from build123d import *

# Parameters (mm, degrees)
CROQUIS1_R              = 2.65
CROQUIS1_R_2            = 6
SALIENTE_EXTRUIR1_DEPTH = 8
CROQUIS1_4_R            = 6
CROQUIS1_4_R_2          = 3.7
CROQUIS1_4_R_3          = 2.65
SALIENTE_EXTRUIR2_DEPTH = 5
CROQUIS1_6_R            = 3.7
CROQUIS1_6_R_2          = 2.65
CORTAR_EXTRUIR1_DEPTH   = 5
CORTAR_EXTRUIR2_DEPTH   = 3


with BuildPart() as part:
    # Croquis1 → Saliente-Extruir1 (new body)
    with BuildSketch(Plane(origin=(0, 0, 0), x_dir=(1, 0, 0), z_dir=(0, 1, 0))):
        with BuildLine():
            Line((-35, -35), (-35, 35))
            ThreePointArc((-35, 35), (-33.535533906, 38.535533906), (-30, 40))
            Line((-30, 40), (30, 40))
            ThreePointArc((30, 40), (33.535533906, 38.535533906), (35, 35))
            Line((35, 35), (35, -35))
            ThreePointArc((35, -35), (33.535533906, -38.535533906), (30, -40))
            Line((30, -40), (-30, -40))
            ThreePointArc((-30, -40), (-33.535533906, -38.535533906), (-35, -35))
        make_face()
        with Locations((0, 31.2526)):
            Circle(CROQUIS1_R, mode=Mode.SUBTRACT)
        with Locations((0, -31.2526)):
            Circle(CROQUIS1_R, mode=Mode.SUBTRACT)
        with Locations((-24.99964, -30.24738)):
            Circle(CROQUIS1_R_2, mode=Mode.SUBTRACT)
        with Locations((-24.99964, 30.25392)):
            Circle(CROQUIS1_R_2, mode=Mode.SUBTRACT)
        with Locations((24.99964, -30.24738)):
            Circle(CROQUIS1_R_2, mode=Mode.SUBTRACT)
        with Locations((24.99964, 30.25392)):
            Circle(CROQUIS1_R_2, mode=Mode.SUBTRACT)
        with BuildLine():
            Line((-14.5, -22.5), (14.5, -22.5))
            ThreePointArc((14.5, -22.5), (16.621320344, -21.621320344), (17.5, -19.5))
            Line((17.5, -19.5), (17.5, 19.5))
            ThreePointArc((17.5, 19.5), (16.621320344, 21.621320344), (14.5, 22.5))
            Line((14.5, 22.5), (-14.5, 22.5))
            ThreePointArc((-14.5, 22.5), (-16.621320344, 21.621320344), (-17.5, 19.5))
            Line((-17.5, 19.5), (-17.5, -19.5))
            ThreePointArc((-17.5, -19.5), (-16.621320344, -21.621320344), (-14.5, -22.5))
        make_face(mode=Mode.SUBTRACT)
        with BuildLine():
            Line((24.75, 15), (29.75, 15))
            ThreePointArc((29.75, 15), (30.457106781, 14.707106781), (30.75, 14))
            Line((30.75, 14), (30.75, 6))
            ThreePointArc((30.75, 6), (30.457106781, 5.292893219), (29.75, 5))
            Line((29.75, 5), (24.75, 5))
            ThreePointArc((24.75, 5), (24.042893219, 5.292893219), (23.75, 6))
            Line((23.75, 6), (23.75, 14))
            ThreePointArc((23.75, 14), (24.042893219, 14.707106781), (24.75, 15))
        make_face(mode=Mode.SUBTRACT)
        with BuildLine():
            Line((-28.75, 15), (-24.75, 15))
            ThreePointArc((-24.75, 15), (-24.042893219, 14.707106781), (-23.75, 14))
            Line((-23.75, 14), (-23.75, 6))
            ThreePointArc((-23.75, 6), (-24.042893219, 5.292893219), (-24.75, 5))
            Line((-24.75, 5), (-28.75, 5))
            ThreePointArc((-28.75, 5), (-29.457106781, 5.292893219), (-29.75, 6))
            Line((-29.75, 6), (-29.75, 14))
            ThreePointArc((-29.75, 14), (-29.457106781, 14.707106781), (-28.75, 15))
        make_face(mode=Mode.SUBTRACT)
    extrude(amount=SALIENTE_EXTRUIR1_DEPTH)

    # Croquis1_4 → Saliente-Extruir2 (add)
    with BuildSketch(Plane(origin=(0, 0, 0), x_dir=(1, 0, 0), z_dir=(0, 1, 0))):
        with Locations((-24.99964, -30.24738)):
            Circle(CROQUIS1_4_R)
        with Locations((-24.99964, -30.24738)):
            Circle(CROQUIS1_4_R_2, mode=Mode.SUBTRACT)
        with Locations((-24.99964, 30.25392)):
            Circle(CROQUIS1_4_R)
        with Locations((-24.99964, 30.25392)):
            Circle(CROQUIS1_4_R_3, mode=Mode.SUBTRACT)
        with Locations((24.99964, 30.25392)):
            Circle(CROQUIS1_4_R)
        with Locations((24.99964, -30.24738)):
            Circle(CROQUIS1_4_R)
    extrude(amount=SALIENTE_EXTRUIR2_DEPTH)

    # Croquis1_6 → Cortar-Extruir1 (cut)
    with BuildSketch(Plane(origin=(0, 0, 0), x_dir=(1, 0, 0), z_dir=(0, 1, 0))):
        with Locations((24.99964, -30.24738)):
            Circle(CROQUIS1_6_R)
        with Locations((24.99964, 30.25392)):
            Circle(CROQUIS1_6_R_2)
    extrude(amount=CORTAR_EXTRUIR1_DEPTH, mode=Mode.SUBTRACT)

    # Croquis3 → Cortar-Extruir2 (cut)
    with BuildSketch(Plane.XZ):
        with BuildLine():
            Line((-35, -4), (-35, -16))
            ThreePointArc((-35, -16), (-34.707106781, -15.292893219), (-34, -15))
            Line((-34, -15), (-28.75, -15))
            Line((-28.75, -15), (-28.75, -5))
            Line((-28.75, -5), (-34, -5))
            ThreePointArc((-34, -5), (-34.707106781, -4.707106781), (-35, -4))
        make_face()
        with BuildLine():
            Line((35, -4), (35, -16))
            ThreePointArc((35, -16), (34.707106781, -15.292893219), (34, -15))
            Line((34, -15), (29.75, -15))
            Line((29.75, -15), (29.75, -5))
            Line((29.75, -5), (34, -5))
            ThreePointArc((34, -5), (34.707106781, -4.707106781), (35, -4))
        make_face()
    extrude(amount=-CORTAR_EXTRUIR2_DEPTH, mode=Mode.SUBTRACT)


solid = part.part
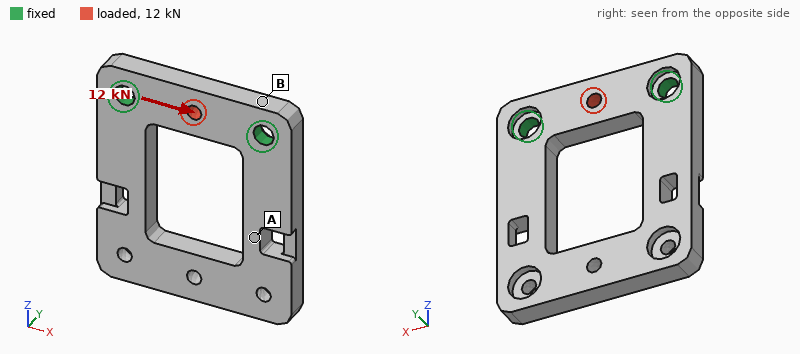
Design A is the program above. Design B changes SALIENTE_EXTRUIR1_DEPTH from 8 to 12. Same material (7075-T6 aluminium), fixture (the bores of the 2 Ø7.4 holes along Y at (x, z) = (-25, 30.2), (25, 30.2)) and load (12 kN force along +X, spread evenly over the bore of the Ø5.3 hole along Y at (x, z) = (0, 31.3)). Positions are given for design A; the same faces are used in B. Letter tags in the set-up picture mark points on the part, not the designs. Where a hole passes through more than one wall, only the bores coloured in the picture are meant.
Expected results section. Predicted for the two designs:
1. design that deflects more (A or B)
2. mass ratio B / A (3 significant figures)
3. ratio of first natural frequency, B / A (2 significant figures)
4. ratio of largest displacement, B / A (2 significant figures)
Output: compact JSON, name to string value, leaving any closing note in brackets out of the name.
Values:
{"design that deflects more": "A", "mass ratio B / A": "1.48", "ratio of first natural frequency, B / A": "1.3", "ratio of largest displacement, B / A": "0.81"}
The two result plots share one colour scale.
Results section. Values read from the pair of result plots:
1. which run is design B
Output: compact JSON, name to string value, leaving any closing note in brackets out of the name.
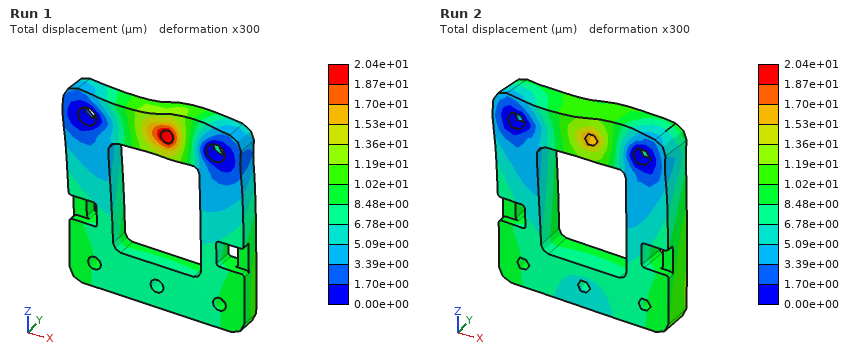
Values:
{"which run is design B": "Run 2"}
